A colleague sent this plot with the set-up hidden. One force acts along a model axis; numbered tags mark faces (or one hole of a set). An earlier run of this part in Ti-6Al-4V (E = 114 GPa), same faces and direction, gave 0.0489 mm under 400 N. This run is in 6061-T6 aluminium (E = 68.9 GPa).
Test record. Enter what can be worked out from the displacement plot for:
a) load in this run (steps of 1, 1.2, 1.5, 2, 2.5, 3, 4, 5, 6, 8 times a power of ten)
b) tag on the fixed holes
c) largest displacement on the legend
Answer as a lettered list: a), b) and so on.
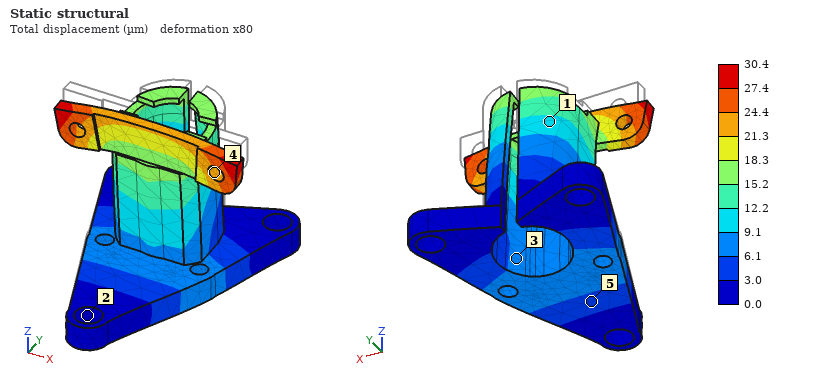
a) 150 N
b) 2
c) 30.4 µm
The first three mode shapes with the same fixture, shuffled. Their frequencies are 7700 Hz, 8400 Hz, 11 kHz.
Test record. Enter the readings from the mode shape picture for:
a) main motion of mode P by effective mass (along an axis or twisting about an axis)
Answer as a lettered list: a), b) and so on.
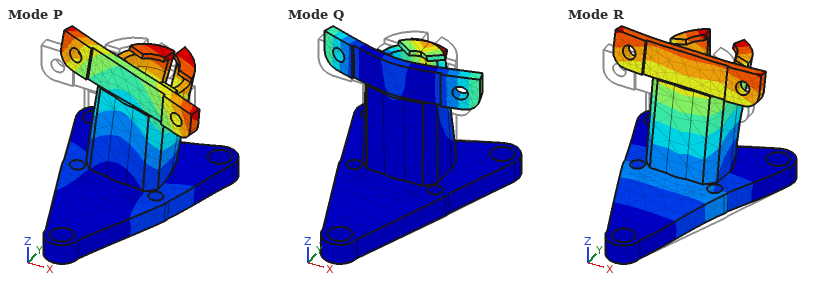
a) along X
